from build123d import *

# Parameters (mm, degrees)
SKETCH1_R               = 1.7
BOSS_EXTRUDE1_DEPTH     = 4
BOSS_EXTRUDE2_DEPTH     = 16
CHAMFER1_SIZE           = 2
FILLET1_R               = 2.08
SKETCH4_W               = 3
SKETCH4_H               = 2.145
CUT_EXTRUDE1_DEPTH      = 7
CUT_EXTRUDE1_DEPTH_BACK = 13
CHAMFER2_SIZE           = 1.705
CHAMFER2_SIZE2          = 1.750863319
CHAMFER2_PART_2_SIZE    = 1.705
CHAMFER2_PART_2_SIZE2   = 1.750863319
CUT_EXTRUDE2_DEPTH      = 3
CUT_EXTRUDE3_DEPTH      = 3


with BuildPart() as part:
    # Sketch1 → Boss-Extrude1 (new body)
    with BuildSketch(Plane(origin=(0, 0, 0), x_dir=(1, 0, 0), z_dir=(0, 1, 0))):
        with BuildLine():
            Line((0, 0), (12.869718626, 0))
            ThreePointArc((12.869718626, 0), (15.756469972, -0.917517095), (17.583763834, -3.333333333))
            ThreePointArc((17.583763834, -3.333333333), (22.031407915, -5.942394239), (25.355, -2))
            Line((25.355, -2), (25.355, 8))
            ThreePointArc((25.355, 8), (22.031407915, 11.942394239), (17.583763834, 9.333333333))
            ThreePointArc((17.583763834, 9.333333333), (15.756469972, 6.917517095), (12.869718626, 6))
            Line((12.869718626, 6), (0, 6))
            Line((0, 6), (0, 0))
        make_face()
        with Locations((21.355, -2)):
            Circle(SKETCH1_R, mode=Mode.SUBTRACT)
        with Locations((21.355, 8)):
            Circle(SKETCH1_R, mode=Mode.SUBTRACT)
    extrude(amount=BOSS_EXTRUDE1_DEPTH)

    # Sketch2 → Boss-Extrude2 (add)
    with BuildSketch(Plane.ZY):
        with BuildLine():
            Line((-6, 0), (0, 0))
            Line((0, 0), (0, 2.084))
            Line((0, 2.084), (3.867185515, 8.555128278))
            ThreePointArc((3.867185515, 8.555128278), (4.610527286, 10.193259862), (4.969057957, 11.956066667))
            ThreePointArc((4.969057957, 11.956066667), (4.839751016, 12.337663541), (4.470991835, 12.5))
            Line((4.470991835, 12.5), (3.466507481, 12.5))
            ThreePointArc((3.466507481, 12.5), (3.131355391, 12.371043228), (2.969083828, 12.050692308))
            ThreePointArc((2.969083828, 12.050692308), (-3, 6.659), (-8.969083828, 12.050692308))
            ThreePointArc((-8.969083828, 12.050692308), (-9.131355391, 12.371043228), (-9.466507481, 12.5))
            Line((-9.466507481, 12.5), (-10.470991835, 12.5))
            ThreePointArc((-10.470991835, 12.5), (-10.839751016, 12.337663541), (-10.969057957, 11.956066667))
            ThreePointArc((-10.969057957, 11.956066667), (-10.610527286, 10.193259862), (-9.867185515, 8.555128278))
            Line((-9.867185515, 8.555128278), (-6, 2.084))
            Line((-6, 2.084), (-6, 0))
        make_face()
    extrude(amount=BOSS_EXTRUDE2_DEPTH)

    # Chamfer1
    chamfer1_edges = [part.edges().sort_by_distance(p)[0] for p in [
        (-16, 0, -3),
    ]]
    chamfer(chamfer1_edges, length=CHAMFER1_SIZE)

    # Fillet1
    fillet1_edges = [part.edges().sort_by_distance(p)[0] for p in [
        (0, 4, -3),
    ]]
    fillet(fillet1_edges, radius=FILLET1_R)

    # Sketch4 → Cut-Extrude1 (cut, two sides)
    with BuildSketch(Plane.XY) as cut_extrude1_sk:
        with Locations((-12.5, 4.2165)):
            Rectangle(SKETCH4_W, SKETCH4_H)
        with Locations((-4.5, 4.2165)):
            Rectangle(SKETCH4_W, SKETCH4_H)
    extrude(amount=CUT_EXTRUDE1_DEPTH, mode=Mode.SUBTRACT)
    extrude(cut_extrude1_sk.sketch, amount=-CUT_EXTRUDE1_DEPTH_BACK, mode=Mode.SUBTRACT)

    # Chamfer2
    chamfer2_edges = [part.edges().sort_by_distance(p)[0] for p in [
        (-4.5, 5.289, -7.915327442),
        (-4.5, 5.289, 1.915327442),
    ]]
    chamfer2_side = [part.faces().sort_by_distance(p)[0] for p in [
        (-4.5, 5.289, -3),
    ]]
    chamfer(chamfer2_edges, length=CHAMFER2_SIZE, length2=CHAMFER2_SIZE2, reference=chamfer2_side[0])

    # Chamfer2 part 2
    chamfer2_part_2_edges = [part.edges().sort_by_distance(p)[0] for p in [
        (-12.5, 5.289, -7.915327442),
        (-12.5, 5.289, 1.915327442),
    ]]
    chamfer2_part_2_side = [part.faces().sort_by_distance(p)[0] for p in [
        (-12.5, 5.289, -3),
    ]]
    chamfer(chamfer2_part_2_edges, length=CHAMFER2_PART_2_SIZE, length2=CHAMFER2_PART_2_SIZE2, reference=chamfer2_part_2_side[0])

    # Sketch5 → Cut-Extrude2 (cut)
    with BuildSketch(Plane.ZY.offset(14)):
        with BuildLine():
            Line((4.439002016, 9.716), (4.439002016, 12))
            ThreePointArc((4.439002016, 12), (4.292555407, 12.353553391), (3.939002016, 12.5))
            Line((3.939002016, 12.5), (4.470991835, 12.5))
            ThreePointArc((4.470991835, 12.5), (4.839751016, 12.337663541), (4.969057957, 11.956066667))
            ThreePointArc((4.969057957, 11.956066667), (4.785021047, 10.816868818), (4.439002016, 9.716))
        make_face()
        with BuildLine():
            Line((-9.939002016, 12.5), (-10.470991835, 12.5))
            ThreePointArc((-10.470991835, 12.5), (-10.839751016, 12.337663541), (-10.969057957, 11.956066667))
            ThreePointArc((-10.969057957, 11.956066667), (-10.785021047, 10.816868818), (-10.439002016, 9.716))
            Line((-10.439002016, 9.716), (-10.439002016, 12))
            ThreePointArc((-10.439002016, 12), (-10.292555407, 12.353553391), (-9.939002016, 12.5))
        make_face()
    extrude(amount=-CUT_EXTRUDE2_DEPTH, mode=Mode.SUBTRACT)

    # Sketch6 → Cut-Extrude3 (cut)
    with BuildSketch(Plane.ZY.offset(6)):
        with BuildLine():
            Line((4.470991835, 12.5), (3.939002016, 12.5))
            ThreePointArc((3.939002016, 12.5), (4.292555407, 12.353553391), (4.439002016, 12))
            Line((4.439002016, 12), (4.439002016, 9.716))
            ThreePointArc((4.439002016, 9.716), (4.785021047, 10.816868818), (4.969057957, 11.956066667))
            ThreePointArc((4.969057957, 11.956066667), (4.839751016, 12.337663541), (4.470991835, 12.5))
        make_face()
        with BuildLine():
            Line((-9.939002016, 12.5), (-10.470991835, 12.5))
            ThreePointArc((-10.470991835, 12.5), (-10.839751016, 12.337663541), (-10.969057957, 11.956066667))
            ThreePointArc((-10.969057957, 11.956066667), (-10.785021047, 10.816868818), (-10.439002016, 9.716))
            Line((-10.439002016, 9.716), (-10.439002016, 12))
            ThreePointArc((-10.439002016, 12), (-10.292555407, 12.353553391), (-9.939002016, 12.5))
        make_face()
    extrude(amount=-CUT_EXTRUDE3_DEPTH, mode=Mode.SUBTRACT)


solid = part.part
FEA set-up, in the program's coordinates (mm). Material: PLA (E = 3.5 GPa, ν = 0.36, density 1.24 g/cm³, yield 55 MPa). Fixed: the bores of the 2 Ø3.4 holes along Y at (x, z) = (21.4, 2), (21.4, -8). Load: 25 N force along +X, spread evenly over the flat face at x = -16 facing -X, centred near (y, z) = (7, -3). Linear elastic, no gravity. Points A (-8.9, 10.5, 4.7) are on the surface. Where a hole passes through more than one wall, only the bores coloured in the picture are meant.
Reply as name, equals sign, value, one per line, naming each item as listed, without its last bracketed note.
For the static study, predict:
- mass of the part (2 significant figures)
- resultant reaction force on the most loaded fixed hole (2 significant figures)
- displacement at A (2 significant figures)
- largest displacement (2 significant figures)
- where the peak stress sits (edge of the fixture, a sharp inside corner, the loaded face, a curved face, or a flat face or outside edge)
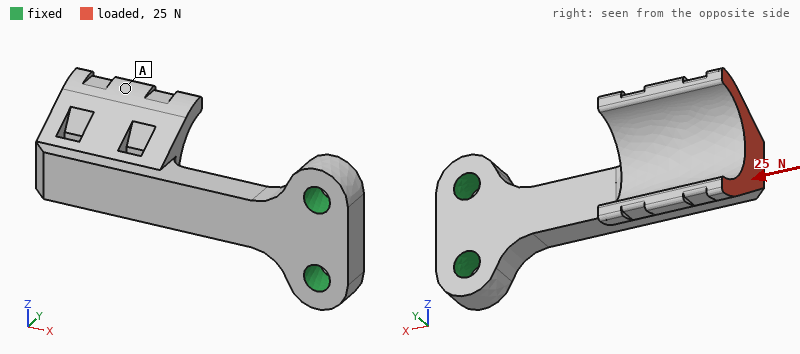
mass of the part = 2.5 g
resultant reaction force on the most loaded fixed hole = 14 N
displacement at A = 0.39 mm
largest displacement = 0.53 mm
where the peak stress sits = a curved face
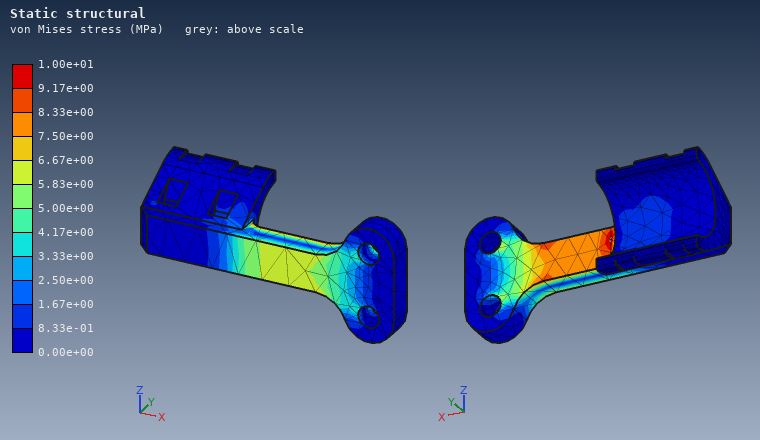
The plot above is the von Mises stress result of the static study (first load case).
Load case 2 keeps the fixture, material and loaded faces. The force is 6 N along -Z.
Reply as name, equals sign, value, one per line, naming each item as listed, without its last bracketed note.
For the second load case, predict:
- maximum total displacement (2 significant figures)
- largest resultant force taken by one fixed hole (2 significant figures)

maximum total displacement = 0.33 mm
largest resultant force taken by one fixed hole = 23 N
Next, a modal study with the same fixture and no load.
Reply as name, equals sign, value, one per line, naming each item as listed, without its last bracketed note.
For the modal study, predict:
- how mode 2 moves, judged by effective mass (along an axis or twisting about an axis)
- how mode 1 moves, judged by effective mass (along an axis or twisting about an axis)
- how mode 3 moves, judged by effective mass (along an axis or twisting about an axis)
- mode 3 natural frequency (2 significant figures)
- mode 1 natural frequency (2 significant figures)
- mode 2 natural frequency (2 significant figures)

how mode 2 moves, judged by effective mass = along Z
how mode 1 moves, judged by effective mass = along Y
how mode 3 moves, judged by effective mass = twisting about X
mode 3 natural frequency = 1900 Hz
mode 1 natural frequency = 520 Hz
mode 2 natural frequency = 830 Hz
